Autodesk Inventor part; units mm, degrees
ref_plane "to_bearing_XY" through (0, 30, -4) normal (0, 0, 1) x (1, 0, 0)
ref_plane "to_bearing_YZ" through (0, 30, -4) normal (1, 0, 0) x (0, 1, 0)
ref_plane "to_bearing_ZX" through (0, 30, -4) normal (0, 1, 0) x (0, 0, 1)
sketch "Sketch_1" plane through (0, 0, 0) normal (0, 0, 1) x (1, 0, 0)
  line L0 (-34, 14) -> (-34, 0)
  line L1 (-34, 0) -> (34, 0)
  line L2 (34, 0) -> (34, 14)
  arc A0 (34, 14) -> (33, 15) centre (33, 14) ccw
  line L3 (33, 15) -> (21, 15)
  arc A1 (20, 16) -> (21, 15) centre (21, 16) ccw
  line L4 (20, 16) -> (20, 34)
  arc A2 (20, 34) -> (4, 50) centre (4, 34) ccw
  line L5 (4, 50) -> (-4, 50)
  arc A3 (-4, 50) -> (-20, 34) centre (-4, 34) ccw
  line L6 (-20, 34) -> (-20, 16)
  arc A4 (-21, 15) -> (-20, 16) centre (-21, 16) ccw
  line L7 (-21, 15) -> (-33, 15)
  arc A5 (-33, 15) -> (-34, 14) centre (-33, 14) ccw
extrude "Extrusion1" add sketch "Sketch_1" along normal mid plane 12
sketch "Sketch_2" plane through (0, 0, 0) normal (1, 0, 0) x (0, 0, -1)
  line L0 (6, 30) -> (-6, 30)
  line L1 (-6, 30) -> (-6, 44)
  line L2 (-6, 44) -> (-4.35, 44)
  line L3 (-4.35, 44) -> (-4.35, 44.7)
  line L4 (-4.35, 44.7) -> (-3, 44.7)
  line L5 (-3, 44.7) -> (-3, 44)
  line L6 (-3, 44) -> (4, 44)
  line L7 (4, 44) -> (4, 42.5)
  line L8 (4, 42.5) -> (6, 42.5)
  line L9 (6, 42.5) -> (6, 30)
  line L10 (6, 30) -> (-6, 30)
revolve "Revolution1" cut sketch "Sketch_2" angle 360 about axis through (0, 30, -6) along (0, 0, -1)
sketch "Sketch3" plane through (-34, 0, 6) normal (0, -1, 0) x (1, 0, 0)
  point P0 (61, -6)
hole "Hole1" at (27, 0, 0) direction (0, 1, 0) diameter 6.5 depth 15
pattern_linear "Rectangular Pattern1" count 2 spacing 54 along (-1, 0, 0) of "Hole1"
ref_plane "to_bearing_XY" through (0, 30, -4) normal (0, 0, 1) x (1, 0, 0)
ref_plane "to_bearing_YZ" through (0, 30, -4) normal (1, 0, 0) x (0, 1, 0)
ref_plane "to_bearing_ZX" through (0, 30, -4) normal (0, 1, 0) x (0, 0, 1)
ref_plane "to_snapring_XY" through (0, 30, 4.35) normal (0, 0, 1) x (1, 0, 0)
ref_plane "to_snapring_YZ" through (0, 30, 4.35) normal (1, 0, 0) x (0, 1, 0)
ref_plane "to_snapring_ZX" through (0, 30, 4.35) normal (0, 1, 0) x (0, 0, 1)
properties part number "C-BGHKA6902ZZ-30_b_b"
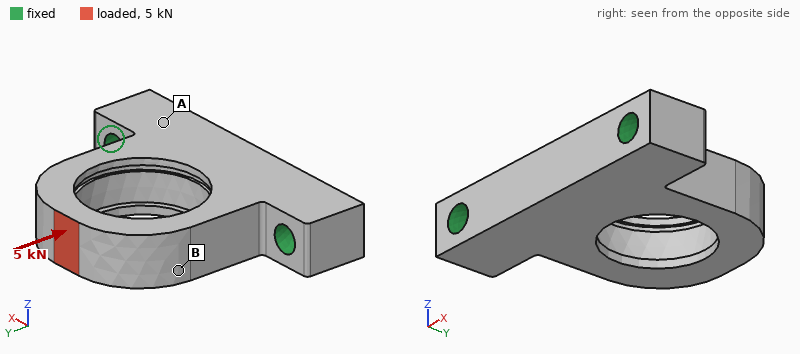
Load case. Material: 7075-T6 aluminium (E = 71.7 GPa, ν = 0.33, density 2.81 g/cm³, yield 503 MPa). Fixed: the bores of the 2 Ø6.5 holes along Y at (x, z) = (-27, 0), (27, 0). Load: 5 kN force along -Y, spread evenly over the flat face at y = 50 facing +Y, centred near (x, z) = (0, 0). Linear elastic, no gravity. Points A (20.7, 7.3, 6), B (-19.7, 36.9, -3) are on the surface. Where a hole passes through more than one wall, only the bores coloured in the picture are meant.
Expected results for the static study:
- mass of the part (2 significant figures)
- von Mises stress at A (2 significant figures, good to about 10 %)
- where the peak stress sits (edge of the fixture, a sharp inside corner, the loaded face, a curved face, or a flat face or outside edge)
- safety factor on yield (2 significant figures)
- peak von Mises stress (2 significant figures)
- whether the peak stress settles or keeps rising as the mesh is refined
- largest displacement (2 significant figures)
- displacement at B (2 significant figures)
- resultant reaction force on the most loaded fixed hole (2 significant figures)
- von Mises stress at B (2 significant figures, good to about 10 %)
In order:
55 g
23 MPa
a curved face
2.0
250 MPa
settles
82 µm
27 µm
2.6 kN
54 MPa
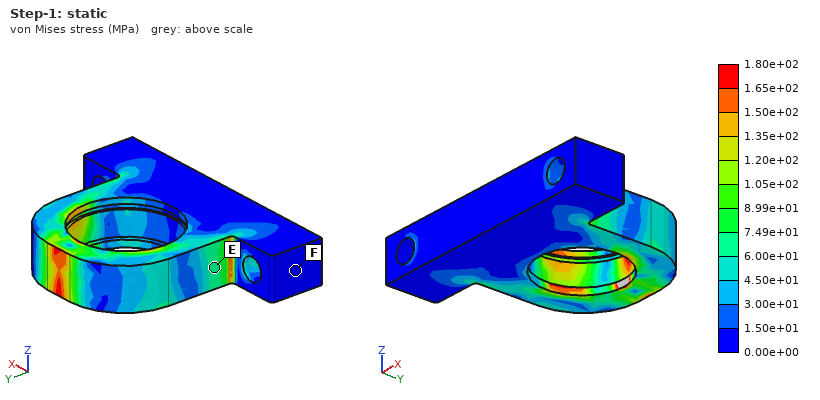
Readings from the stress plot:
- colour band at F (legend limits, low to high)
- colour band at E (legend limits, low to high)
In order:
0.00e+00 to 1.50e+01 MPa
6.00e+01 to 7.49e+01 MPa
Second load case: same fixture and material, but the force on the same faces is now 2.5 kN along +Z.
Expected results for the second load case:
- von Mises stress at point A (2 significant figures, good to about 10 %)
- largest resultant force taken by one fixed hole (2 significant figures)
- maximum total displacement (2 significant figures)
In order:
150 MPa
1.3 kN
0.51 mm
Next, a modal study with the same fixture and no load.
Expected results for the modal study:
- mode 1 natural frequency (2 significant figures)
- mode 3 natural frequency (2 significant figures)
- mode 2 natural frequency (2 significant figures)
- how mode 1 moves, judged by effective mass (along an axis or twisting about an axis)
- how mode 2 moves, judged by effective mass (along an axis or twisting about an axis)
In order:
4200 Hz
10 kHz
7800 Hz
along Z
along X
